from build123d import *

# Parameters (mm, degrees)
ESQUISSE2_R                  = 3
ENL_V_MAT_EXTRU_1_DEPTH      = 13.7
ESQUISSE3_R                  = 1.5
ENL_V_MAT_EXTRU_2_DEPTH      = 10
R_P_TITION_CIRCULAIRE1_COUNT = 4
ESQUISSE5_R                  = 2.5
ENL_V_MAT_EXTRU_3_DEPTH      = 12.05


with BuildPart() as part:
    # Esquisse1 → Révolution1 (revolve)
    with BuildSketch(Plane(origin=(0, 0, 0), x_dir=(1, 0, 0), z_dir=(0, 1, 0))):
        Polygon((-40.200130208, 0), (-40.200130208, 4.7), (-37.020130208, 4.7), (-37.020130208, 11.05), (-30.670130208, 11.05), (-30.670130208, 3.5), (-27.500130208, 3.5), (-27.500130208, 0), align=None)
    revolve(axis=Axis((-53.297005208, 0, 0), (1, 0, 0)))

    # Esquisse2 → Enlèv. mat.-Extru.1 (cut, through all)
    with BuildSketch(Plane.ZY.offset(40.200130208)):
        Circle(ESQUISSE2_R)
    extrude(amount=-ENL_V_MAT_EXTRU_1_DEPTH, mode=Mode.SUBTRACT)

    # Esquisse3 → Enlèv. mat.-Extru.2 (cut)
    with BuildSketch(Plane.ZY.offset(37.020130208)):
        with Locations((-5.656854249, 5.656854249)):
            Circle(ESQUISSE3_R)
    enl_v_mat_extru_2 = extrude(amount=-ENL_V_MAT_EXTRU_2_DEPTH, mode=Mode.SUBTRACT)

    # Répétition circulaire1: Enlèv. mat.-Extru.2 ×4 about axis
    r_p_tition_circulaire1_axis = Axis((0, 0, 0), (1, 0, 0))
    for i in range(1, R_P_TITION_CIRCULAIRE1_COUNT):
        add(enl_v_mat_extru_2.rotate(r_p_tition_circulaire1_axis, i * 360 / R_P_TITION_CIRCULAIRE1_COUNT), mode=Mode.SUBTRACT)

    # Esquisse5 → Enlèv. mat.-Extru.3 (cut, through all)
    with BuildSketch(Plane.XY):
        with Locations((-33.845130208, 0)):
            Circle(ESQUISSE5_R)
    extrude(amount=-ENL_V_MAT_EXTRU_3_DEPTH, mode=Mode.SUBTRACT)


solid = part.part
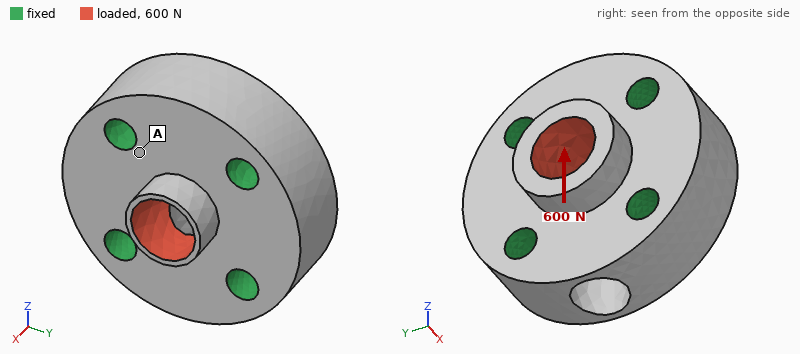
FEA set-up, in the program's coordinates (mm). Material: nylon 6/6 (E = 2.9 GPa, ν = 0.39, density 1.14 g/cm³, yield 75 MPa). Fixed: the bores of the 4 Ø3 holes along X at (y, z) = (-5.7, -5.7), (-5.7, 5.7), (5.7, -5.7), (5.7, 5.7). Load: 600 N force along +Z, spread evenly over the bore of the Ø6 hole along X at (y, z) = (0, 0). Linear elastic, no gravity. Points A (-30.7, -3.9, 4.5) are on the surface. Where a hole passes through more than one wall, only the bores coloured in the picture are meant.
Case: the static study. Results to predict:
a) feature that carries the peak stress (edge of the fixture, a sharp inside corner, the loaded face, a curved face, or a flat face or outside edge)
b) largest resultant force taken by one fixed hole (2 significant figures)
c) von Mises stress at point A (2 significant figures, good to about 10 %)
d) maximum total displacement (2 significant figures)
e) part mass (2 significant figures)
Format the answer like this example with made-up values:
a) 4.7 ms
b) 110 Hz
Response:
a) the loaded face
b) 170 N
c) 6.2 MPa
d) 0.11 mm
e) 2.4 g
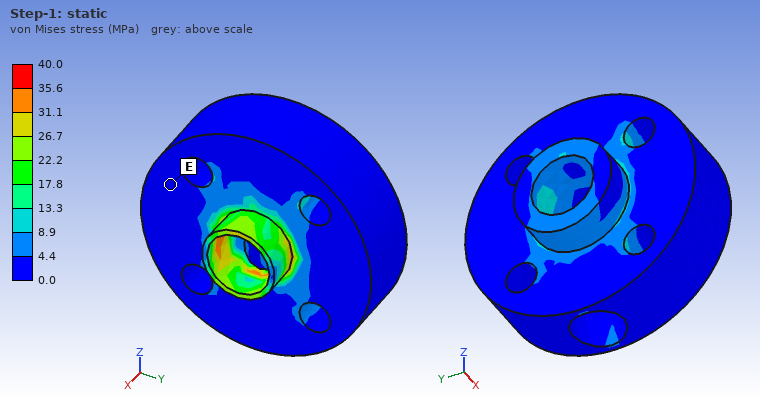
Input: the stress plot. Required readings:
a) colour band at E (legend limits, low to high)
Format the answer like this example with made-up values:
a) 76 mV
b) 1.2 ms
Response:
a) 0.0 to 4.4 MPa
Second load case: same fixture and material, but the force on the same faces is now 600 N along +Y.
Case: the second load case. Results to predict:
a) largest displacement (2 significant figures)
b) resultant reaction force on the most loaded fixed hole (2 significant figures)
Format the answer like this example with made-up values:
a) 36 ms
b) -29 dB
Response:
a) 98 µm
b) 180 N
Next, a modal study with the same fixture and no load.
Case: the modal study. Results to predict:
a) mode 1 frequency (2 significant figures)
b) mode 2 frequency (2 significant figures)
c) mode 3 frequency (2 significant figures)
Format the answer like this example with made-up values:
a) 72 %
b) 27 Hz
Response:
a) 31 kHz
b) 33 kHz
c) 33 kHz
